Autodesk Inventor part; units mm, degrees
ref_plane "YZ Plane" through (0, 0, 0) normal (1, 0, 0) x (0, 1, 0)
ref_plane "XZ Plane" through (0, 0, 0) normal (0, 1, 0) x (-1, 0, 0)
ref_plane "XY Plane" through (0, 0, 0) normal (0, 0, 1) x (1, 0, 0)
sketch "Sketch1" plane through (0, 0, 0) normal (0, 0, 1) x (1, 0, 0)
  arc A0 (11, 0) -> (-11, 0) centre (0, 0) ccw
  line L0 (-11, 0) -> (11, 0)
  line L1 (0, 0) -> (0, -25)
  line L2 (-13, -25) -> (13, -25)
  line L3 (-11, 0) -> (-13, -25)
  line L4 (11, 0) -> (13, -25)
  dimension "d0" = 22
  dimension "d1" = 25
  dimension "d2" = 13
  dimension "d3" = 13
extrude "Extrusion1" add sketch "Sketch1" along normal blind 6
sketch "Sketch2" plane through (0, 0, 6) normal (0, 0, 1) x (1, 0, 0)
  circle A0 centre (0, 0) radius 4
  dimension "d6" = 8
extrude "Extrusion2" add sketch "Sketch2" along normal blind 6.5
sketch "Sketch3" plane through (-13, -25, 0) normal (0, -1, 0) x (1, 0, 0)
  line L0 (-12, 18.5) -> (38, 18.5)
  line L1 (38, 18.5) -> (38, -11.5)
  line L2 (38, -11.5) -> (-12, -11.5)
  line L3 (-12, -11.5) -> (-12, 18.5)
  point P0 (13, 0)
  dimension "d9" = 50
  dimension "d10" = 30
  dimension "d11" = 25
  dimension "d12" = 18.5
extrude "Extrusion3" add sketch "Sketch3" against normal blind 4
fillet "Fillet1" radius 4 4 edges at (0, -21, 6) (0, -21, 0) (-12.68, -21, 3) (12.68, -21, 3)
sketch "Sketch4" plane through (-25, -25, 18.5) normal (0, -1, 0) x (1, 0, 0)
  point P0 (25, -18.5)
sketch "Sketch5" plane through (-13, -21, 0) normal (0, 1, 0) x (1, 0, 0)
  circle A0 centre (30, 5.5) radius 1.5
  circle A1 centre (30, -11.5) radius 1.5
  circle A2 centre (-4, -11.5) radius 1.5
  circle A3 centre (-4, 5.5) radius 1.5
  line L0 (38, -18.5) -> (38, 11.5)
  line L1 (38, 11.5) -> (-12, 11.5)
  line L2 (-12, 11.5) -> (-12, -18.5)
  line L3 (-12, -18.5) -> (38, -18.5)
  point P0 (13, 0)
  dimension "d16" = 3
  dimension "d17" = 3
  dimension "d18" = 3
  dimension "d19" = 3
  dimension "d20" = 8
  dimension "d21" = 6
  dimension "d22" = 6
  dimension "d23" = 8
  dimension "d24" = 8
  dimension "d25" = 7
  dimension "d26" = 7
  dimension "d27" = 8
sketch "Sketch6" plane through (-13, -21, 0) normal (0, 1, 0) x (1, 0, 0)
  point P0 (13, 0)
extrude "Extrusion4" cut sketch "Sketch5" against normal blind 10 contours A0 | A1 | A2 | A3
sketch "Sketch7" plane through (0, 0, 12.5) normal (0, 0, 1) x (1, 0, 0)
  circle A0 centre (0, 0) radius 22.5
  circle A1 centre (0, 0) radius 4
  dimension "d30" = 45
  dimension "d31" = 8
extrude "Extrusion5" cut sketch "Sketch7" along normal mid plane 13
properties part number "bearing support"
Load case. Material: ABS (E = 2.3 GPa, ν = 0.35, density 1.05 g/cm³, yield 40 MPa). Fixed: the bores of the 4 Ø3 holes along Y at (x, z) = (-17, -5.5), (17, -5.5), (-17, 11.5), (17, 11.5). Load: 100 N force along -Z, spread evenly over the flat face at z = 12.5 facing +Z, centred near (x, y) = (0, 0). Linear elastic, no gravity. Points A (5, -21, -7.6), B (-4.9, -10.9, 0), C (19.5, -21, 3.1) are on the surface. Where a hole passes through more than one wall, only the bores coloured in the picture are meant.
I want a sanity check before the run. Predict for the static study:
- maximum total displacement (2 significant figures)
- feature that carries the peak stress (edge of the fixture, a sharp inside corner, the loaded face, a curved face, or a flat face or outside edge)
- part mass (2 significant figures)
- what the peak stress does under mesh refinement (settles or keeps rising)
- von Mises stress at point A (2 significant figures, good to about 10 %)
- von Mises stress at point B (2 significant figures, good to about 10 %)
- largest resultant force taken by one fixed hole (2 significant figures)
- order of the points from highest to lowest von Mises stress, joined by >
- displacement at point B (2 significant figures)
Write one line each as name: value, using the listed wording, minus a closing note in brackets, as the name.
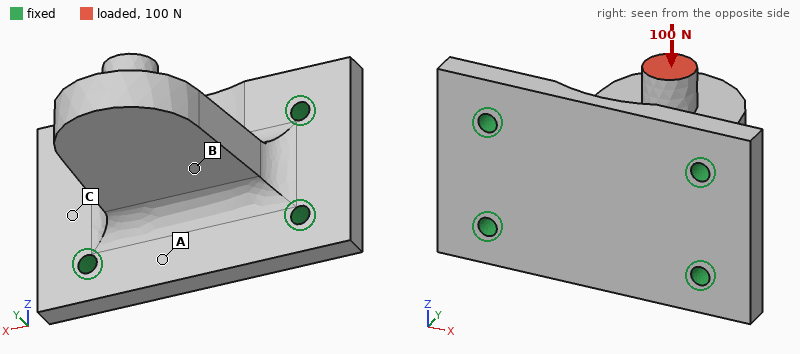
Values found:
maximum total displacement: 0.81 mm
feature that carries the peak stress: a sharp inside corner
part mass: 11 g
what the peak stress does under mesh refinement: keeps rising
von Mises stress at point A: 3.2 MPa
von Mises stress at point B: 7.6 MPa
largest resultant force taken by one fixed hole: 78 N
order of the points from highest to lowest von Mises stress, joined by >: B > A > C
displacement at point B: 0.19 mm
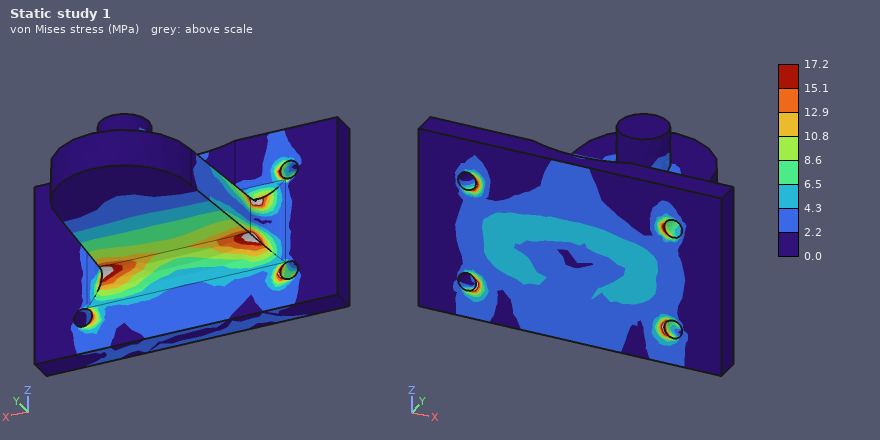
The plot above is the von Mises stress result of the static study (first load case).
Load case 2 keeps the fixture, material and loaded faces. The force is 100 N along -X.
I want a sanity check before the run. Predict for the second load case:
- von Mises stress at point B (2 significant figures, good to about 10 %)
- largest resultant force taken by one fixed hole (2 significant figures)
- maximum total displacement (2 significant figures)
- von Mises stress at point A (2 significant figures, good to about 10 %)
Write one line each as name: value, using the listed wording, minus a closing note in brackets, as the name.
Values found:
von Mises stress at point B: 3.6 MPa
largest resultant force taken by one fixed hole: 67 N
maximum total displacement: 0.24 mm
von Mises stress at point A: 1.1 MPa
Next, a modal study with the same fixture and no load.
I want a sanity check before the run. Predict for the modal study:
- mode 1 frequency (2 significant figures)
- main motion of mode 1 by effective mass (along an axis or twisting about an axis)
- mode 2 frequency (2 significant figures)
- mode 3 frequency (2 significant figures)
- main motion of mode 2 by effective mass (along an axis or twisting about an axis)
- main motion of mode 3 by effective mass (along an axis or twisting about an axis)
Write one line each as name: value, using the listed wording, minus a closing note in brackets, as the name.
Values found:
mode 1 frequency: 1300 Hz
main motion of mode 1 by effective mass: along Z
mode 2 frequency: 3300 Hz
mode 3 frequency: 4300 Hz
main motion of mode 2 by effective mass: along X
main motion of mode 3 by effective mass: along Y
